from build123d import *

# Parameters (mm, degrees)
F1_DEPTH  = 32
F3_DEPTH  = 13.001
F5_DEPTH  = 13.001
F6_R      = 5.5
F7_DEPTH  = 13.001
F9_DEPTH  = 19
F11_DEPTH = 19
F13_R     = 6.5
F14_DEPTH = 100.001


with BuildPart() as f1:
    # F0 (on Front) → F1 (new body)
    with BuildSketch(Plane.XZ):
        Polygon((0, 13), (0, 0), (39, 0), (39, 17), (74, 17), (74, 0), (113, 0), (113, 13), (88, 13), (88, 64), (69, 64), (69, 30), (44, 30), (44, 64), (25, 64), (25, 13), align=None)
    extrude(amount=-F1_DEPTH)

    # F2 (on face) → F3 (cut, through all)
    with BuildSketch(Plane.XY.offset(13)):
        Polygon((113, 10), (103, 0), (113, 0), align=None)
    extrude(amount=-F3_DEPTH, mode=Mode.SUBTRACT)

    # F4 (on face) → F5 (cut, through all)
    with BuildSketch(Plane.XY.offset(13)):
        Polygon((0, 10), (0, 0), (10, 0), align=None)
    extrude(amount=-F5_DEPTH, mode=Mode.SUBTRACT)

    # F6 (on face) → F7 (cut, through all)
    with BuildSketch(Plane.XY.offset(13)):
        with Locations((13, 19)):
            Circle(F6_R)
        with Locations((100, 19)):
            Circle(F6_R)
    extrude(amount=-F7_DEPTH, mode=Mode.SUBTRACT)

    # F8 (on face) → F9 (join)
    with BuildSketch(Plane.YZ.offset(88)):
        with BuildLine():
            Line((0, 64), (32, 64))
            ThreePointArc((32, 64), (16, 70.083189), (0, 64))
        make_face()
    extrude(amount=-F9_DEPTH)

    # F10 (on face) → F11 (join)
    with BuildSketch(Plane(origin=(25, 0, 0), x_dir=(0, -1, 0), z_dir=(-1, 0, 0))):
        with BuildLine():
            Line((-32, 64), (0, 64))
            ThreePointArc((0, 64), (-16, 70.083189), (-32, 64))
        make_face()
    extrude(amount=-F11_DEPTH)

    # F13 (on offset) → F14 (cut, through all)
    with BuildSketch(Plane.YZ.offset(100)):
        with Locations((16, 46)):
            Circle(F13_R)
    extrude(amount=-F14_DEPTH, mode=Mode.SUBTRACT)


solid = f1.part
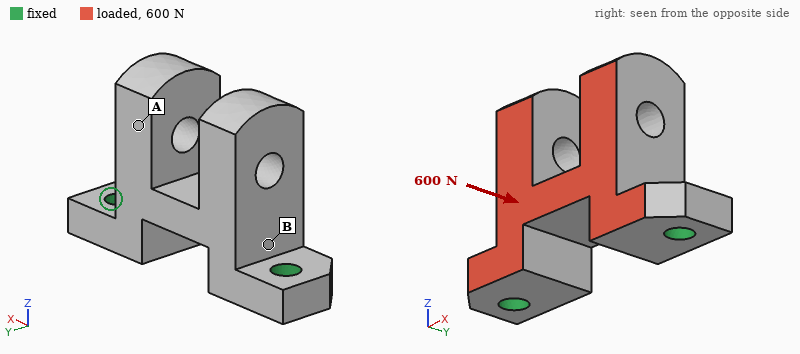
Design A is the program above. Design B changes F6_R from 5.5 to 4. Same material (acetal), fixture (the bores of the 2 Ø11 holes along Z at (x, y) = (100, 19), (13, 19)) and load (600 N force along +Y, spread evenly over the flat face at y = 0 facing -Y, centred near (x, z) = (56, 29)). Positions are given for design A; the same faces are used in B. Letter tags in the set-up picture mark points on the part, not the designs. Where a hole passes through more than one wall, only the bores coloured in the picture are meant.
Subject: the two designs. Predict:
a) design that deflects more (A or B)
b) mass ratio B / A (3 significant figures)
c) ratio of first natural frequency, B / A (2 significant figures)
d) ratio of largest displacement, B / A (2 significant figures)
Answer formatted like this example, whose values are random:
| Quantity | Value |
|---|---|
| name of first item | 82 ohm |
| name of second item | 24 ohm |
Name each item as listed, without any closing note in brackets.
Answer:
| Quantity | Value |
|---|---|
| design that deflects more | B |
| mass ratio B / A | 1.01 |
| ratio of first natural frequency, B / A | 0.90 |
| ratio of largest displacement, B / A | 1.2 |
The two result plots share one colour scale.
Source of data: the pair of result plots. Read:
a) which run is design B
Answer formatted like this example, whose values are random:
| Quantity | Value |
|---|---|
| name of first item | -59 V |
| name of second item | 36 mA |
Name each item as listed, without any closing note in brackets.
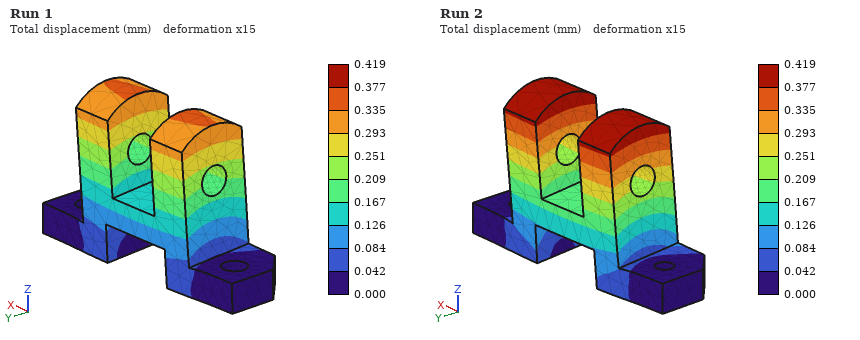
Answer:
| Quantity | Value |
|---|---|
| which run is design B | Run 2 |
